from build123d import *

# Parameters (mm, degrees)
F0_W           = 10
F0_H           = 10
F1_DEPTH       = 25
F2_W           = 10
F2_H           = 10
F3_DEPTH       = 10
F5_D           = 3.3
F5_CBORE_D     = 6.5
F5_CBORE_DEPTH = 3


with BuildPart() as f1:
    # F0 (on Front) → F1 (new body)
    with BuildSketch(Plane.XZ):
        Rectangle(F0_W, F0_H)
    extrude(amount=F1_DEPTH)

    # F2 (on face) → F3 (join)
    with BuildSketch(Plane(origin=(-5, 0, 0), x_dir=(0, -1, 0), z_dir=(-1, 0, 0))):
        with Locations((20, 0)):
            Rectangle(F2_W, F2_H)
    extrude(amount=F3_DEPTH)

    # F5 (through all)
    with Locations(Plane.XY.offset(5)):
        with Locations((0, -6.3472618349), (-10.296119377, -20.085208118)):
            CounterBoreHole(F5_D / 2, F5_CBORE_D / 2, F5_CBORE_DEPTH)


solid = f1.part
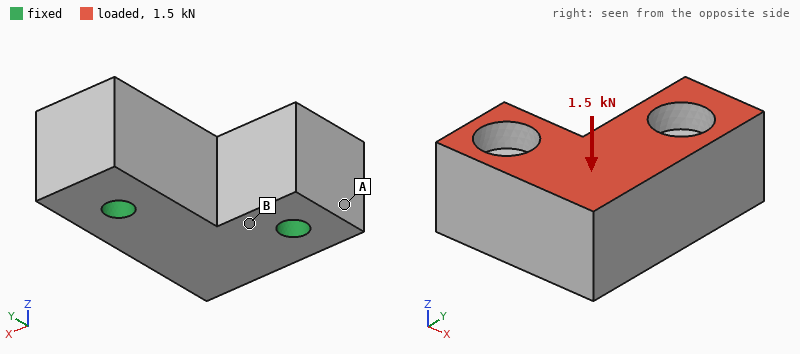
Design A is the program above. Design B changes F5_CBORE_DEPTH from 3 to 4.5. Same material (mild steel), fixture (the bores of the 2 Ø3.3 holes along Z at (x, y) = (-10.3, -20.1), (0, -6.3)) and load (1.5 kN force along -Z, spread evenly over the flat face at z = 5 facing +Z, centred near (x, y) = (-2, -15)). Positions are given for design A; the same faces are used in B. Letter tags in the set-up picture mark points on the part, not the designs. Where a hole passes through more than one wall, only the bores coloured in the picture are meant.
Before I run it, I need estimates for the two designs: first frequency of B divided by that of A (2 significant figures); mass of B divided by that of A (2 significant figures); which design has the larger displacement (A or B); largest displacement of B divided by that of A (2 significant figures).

0.82
0.98
B
1.4
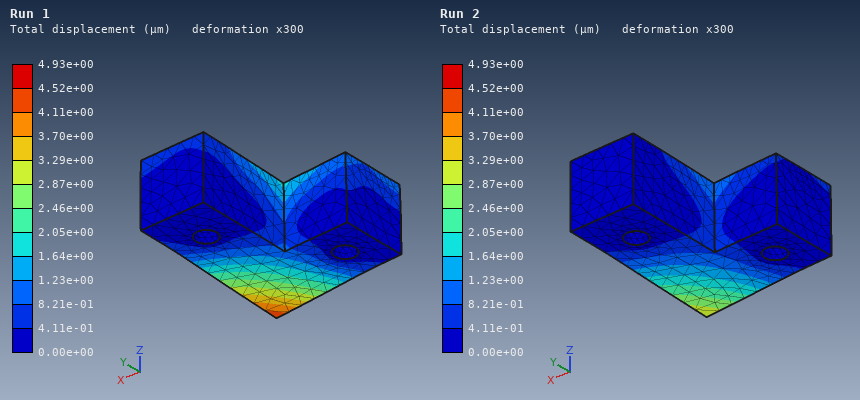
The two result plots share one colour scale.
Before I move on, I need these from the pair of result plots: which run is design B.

Run 1
